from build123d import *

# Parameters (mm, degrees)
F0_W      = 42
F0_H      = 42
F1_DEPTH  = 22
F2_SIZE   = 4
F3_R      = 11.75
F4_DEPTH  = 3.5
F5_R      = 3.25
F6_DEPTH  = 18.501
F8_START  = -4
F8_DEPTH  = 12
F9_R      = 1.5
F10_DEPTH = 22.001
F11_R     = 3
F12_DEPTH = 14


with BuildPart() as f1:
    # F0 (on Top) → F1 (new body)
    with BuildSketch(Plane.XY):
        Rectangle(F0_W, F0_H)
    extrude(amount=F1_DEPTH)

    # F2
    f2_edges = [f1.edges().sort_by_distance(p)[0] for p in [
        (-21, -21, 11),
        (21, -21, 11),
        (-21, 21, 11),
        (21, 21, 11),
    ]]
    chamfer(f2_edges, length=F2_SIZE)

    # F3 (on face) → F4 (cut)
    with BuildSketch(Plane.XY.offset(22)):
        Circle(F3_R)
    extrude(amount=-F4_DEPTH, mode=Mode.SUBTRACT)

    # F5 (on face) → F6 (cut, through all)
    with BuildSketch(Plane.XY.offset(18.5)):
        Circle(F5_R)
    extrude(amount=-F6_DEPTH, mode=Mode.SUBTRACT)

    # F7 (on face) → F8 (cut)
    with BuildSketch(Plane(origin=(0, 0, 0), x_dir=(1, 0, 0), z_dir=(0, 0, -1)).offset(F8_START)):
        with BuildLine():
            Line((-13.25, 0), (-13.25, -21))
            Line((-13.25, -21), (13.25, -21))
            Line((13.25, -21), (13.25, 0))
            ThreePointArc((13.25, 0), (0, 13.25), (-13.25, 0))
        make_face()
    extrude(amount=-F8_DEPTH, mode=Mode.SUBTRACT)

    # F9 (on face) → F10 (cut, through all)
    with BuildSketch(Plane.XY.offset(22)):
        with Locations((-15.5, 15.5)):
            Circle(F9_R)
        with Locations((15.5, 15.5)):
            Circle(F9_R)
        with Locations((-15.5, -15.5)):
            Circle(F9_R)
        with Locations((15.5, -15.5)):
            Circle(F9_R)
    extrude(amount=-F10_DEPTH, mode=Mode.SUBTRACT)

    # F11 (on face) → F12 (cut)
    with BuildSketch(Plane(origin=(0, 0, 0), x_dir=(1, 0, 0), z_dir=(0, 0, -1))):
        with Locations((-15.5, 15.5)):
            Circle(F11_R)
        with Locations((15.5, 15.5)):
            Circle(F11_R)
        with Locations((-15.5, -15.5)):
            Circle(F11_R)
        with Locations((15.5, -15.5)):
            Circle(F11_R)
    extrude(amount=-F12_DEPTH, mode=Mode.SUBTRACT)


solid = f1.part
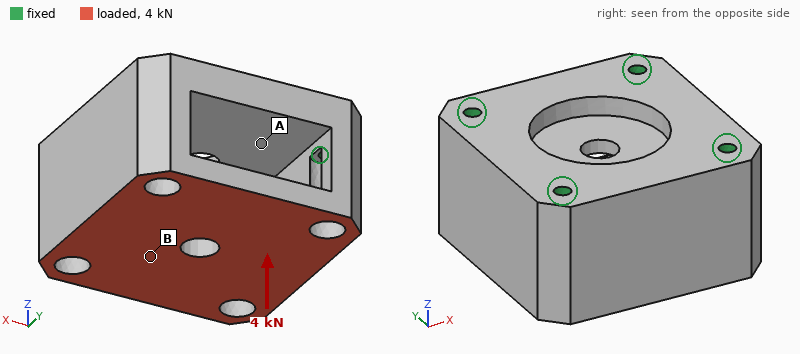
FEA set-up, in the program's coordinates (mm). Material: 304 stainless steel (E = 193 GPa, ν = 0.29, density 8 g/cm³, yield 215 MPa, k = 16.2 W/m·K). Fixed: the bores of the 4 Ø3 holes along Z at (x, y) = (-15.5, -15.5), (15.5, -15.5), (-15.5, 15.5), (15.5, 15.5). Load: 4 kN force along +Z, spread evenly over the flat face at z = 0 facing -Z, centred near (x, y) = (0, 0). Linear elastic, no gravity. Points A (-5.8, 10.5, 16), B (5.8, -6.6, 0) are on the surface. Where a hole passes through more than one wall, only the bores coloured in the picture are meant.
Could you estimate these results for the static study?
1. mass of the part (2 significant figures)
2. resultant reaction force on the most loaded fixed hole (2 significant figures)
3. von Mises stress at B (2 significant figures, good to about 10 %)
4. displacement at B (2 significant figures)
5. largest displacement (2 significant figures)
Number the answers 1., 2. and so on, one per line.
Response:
1. 200 g
2. 1.1 kN
3. 16 MPa
4. 3.0 µm
5. 12 µm
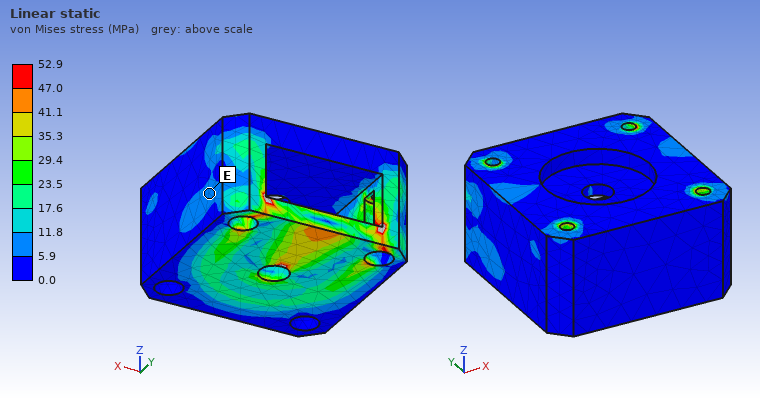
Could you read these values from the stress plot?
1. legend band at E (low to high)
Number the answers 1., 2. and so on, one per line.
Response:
1. 5.9 to 11.8 MPa
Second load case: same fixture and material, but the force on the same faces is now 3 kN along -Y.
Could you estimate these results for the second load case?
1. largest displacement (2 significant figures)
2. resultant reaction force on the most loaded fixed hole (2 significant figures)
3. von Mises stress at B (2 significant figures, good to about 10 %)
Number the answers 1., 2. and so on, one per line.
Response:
1. 4.5 µm
2. 1.1 kN
3. 7.6 MPa
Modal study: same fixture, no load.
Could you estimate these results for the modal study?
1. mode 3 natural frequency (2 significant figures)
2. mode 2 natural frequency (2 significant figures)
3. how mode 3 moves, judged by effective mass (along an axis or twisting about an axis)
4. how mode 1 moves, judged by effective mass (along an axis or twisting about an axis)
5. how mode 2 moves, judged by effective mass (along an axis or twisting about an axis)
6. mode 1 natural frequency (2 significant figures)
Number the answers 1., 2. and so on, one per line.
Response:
1. 21 kHz
2. 17 kHz
3. along Y
4. along X
5. along Z
6. 15 kHz
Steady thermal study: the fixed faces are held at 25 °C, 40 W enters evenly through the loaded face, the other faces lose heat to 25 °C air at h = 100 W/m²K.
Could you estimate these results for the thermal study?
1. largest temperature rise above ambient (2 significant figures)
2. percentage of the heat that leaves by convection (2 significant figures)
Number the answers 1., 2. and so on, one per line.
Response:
1. 77 K
2. 50 %
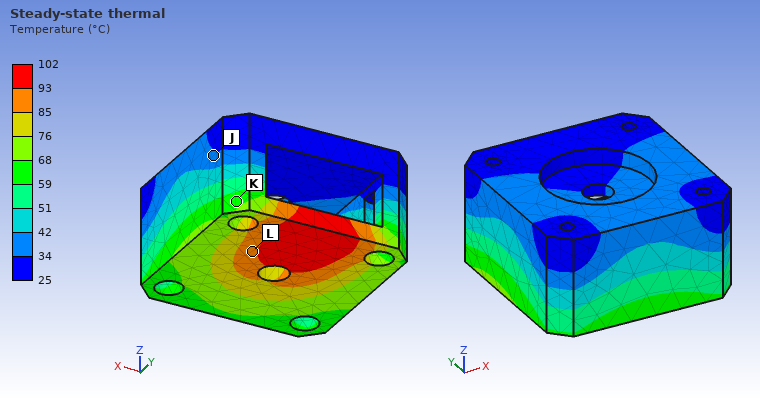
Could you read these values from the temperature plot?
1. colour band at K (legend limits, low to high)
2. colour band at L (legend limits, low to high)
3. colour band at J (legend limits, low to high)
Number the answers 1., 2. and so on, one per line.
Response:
1. 59 to 68 °C
2. 85 to 93 °C
3. 34 to 42 °C
